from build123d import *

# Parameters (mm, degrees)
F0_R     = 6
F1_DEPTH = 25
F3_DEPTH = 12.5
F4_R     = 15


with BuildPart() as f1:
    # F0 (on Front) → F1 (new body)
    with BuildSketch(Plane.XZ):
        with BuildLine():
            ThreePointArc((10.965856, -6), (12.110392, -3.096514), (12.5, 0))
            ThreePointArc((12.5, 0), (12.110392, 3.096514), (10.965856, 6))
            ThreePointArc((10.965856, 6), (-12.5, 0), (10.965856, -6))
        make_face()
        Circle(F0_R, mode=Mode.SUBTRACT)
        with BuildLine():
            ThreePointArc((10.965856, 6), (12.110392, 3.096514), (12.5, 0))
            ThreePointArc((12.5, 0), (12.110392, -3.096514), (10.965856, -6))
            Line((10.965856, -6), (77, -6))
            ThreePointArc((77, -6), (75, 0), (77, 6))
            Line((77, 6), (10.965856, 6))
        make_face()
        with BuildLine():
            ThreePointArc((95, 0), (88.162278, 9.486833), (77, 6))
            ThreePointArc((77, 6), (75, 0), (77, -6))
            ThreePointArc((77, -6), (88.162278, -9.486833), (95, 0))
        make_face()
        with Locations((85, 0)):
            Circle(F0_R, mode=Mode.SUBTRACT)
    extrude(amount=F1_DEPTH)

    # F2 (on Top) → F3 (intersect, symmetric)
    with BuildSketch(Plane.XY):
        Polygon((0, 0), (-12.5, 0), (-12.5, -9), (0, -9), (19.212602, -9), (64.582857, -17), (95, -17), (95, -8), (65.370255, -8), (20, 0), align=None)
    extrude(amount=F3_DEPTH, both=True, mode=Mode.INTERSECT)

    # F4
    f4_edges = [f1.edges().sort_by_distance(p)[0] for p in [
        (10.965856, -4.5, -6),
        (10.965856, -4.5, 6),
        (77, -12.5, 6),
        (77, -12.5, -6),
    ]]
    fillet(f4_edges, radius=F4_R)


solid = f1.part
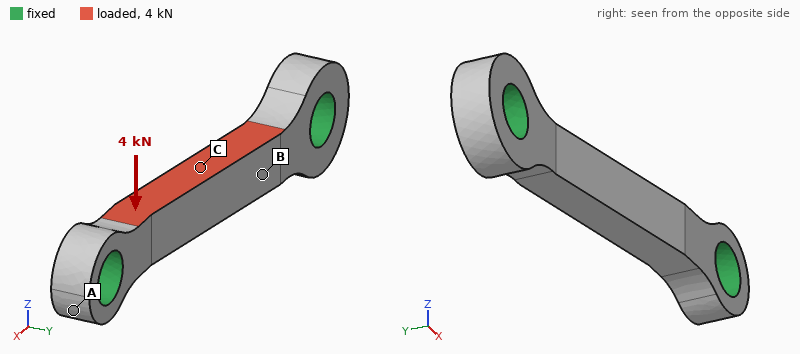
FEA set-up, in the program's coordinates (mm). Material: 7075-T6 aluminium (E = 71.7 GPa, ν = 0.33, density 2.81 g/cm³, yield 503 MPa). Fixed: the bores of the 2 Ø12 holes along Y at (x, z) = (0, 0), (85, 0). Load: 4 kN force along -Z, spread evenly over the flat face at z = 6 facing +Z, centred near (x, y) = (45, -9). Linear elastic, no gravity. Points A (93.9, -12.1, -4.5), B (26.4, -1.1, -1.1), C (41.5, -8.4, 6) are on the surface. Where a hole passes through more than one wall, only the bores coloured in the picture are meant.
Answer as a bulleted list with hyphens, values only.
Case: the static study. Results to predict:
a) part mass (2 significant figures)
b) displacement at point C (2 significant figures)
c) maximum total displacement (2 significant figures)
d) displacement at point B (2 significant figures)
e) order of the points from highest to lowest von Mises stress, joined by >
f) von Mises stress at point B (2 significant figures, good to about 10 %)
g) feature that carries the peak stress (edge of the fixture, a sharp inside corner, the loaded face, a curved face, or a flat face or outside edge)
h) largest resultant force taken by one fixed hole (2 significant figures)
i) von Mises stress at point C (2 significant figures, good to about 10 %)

- 35 g
- 68 µm
- 70 µm
- 41 µm
- C > B > A
- 32 MPa
- a curved face
- 2.1 kN
- 69 MPa
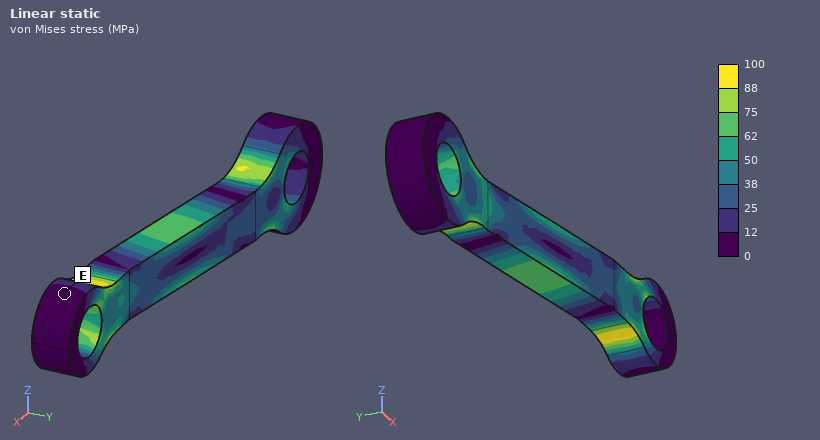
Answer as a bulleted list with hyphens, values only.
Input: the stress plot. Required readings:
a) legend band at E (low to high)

- 0 to 12 MPa
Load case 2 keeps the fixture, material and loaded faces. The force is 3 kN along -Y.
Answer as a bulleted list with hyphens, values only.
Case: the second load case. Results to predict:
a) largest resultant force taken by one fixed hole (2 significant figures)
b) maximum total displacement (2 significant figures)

- 1.6 kN
- 0.12 mm
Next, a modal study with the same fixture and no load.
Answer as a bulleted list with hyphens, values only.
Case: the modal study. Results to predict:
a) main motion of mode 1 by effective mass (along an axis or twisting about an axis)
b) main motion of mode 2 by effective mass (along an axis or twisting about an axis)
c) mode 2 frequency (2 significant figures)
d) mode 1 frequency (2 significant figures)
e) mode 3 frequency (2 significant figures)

- along Y
- along Z
- 10 kHz
- 7900 Hz
- 19 kHz
